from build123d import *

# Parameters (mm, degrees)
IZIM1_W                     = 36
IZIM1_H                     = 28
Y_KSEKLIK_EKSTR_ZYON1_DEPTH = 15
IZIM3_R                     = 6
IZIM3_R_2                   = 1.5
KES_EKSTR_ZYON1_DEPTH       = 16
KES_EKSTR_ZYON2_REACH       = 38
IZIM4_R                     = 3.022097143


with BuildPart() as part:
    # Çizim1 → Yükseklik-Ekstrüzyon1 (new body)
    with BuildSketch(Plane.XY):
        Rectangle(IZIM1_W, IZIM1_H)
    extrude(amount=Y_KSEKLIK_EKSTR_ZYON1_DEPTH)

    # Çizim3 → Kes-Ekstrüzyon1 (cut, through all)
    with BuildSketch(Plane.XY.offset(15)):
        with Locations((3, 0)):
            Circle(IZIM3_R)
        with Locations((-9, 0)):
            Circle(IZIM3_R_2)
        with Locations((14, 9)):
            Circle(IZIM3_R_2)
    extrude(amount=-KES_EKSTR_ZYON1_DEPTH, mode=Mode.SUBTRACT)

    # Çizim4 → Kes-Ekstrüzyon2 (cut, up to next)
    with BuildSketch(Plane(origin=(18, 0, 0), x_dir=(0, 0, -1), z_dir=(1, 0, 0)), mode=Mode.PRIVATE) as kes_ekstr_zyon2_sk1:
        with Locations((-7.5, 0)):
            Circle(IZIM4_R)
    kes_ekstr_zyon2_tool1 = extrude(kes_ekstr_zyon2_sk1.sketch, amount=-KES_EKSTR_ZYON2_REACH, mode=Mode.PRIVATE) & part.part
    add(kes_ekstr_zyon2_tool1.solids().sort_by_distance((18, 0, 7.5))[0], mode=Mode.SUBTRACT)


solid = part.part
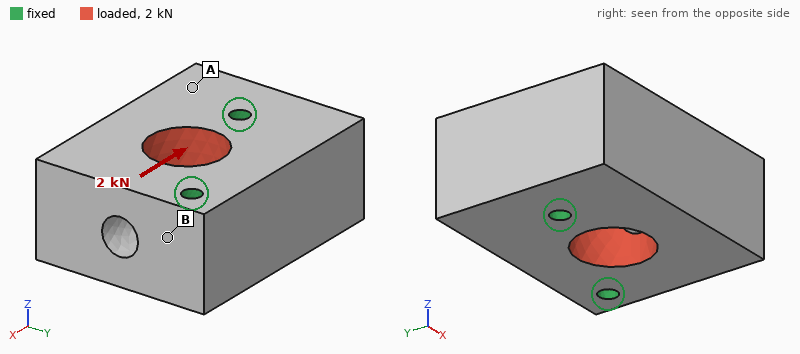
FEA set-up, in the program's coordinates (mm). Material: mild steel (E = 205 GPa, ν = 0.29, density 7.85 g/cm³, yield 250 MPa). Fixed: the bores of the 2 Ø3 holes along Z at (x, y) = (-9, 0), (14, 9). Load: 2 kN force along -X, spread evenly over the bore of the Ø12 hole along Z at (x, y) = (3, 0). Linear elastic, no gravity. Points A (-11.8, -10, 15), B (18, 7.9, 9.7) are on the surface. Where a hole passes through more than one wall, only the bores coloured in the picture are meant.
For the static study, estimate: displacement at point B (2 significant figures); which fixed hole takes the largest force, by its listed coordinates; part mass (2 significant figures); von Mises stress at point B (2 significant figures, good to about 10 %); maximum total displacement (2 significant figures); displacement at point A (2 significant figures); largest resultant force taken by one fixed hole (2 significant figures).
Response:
0.15 µm
(-9, 0)
100 g
5.8 MPa
0.87 µm
0.52 µm
1.3 kN
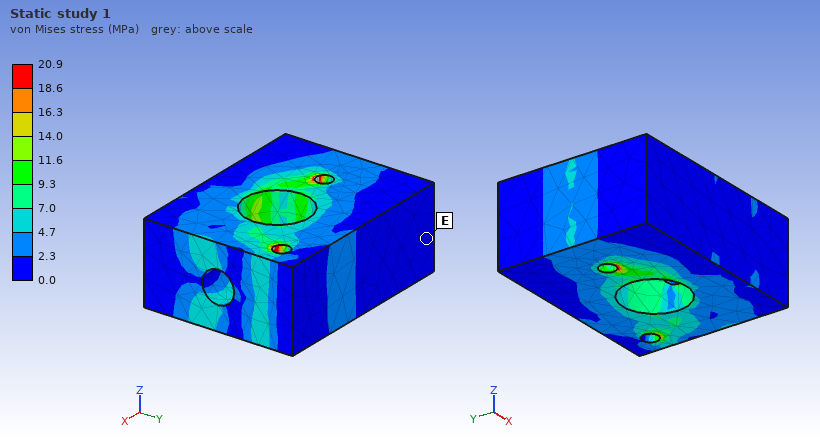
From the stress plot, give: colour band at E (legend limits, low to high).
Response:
0.0 to 2.3 MPa
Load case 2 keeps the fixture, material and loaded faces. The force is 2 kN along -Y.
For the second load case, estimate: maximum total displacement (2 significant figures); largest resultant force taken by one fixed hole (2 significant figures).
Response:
0.71 µm
1.0 kN
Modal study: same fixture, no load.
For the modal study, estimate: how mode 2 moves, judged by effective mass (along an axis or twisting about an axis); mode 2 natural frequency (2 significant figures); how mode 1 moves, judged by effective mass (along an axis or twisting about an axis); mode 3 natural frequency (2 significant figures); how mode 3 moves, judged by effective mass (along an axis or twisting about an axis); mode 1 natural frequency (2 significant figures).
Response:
along X
25 kHz
along Z
32 kHz
twisting about X
18 kHz
